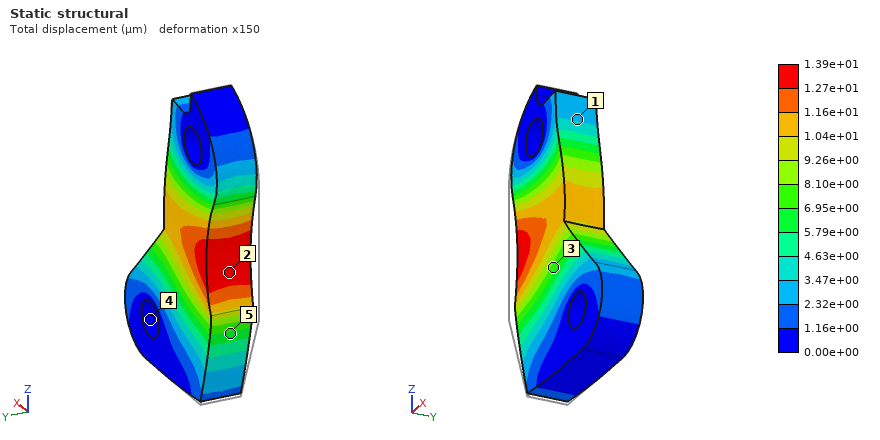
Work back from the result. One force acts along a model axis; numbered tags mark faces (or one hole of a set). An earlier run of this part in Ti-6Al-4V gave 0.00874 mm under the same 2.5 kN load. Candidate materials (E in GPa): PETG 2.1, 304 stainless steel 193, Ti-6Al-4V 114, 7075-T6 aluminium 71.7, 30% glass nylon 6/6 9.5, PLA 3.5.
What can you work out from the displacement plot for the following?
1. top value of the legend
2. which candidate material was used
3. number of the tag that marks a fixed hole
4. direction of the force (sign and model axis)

1.39e+01 µm
7075-T6 aluminium
4
+X
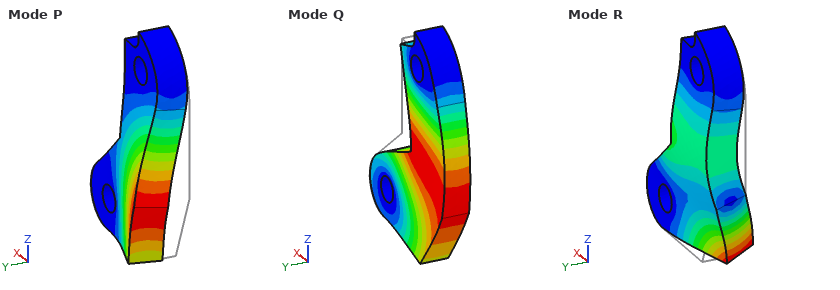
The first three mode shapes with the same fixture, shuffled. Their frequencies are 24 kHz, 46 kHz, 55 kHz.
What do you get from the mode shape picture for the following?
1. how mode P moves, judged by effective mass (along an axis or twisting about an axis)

along Y
